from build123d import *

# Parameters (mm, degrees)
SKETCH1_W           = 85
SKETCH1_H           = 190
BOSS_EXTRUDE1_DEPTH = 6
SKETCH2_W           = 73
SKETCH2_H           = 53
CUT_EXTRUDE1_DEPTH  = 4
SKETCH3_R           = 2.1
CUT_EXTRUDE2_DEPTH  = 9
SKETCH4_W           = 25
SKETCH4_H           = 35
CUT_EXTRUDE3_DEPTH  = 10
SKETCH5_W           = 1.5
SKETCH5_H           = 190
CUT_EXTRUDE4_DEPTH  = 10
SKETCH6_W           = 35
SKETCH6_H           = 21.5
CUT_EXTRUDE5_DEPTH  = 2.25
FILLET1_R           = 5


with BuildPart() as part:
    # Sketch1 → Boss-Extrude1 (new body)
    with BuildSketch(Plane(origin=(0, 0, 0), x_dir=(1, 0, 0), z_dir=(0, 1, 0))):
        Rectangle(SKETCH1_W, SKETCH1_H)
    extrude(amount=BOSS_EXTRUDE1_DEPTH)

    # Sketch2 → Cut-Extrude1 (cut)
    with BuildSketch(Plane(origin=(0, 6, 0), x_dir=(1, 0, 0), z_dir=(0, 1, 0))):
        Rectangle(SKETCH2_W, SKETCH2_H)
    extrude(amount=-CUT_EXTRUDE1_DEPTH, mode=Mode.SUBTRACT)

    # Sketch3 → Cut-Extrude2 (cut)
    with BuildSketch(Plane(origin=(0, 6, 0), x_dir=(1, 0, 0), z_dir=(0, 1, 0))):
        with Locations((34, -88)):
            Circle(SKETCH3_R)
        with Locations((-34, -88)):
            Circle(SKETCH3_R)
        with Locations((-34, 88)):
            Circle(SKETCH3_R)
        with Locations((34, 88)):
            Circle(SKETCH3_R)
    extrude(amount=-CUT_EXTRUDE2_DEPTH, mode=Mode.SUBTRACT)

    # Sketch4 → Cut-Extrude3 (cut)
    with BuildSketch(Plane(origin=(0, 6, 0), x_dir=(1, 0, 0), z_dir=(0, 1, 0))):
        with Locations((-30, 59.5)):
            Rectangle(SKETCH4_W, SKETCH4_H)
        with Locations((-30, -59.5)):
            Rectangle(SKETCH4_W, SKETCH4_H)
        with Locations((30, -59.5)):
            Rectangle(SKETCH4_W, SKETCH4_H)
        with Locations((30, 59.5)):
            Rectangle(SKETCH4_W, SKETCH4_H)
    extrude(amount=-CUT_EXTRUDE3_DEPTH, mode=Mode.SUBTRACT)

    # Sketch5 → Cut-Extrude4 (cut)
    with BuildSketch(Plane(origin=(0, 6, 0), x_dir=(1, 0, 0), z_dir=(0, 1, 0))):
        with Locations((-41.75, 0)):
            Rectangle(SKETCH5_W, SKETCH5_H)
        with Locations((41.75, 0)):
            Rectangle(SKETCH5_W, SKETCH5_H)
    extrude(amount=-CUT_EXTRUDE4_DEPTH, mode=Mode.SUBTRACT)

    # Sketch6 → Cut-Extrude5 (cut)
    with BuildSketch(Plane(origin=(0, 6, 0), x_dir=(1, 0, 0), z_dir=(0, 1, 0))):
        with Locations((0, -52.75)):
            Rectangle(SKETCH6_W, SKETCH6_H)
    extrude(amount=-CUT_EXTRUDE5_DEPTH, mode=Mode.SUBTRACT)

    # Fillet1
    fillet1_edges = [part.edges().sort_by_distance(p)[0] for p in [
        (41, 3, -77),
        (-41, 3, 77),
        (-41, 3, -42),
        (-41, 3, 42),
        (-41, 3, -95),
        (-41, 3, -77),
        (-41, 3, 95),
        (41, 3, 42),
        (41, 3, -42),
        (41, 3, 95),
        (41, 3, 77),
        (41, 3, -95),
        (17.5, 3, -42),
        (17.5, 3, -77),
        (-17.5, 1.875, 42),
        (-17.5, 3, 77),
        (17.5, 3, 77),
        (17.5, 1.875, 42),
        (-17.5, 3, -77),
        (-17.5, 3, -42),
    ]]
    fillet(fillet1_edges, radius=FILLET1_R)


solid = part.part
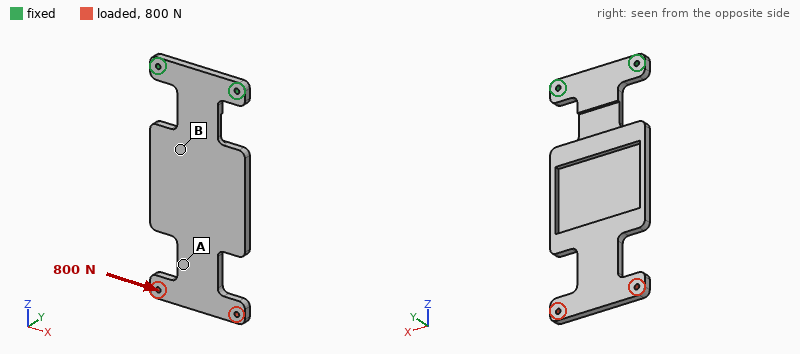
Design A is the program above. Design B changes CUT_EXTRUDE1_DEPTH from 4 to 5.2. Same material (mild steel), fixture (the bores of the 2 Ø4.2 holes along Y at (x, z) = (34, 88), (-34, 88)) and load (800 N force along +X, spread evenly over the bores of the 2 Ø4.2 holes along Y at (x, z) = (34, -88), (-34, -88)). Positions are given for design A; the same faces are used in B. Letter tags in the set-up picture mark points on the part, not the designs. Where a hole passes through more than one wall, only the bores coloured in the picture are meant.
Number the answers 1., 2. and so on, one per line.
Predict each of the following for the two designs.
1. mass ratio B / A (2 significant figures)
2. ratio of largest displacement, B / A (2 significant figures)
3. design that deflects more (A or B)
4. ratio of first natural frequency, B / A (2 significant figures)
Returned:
1. 0.92
2. 1.1
3. B
4. 1.00
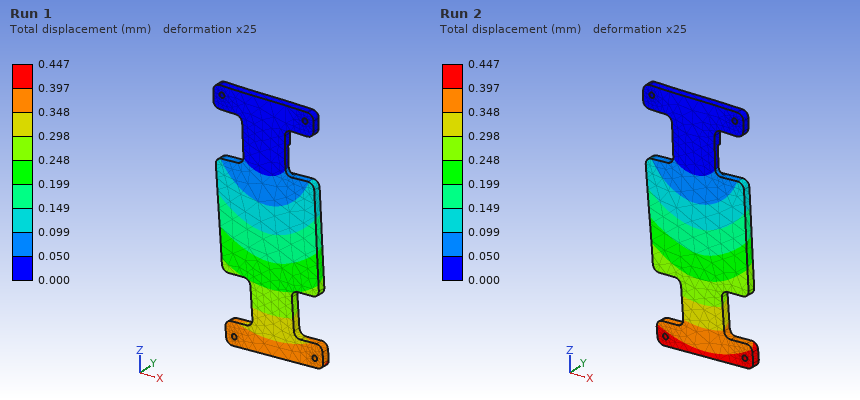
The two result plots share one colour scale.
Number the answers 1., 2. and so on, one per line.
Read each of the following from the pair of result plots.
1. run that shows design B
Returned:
1. Run 2
